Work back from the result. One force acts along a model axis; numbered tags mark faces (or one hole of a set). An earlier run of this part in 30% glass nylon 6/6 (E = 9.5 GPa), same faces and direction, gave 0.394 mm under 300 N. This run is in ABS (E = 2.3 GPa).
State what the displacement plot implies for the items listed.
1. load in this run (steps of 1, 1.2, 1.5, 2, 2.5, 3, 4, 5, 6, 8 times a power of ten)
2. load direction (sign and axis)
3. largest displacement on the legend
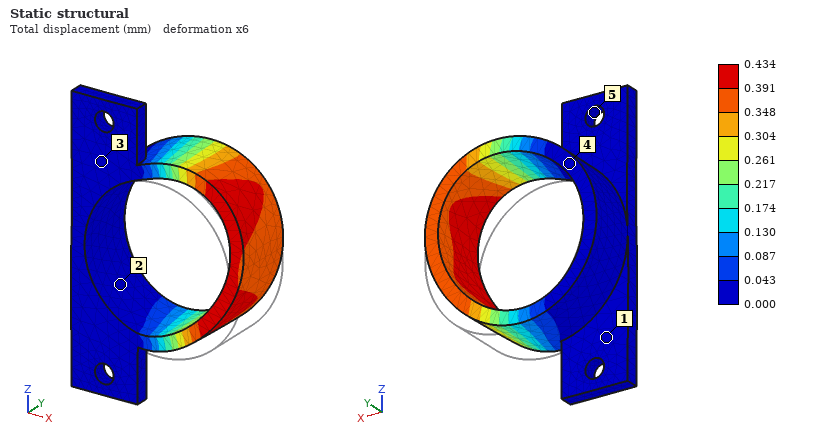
80 N
+Z
0.434 mm
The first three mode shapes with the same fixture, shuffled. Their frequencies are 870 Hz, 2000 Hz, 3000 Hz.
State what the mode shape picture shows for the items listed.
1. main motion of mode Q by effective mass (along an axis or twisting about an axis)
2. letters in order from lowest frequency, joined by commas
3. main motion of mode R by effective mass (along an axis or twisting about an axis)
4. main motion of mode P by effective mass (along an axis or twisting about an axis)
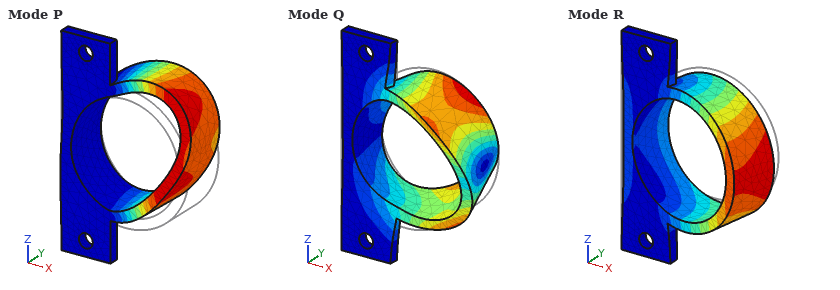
twisting about X
R, P, Q
along Y
along Z
